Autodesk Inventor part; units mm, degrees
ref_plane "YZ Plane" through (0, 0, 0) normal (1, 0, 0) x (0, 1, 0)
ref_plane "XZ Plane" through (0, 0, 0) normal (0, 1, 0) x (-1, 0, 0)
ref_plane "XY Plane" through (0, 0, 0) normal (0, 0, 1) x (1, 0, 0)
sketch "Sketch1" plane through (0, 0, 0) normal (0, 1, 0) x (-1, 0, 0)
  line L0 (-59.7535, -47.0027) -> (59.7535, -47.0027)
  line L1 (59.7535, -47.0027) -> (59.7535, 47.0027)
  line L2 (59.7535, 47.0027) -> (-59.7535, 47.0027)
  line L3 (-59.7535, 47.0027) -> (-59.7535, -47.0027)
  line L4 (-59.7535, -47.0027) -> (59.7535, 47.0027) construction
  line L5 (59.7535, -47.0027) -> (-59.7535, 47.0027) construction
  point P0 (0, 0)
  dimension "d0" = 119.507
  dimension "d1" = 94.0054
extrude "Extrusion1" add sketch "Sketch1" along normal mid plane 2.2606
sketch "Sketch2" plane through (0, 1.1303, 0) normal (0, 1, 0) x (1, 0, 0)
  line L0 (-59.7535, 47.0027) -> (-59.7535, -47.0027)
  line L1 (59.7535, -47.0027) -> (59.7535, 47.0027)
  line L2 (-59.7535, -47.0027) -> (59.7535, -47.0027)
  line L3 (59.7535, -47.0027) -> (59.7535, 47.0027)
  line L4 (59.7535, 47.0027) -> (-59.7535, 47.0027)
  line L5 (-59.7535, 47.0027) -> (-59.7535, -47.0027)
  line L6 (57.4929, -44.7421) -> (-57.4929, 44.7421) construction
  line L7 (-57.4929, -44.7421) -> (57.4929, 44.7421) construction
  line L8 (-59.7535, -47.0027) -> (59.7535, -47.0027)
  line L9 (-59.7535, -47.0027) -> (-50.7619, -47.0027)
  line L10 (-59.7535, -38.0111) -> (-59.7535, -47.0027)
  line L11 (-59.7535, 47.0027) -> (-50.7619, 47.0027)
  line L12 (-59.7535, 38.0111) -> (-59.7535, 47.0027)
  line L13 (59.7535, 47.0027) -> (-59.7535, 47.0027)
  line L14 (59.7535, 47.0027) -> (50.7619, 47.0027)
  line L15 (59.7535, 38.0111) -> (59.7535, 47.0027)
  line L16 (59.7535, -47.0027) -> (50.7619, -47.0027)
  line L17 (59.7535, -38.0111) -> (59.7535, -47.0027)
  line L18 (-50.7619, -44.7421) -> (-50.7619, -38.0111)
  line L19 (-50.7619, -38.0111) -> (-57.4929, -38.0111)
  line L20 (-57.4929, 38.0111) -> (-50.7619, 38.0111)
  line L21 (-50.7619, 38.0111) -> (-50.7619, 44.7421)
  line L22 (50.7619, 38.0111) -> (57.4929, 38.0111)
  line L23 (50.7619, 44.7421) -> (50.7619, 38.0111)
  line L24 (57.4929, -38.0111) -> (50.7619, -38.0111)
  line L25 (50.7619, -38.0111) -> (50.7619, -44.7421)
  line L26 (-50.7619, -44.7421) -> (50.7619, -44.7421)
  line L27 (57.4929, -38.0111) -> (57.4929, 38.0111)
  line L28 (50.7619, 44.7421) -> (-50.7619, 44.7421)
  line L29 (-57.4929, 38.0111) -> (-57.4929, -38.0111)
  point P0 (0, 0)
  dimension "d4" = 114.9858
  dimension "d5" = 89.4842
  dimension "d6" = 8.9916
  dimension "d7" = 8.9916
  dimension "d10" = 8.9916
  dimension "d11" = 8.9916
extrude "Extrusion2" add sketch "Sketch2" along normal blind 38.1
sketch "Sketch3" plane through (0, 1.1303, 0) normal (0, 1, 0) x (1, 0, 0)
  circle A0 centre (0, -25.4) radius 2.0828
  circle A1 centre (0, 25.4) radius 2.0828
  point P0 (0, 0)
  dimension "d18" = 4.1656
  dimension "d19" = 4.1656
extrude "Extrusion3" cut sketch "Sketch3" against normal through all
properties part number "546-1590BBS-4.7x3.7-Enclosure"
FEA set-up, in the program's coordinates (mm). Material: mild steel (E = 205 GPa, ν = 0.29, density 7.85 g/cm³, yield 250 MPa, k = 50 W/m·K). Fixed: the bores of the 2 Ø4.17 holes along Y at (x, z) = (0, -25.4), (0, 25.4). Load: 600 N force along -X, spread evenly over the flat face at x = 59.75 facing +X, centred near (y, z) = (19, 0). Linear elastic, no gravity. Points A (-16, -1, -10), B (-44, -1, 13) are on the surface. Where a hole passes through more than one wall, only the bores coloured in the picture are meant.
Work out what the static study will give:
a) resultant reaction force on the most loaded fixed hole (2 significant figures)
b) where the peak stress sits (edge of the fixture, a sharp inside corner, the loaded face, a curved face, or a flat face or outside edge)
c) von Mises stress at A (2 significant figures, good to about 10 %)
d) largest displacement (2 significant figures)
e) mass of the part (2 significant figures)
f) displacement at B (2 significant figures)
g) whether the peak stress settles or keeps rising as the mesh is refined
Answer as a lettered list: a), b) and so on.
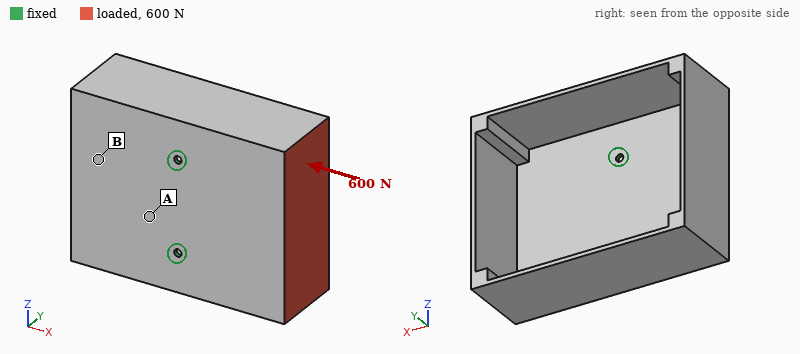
a) 300 N
b) edge of the fixture
c) 31 MPa
d) 0.42 mm
e) 540 g
f) 0.21 mm
g) keeps rising
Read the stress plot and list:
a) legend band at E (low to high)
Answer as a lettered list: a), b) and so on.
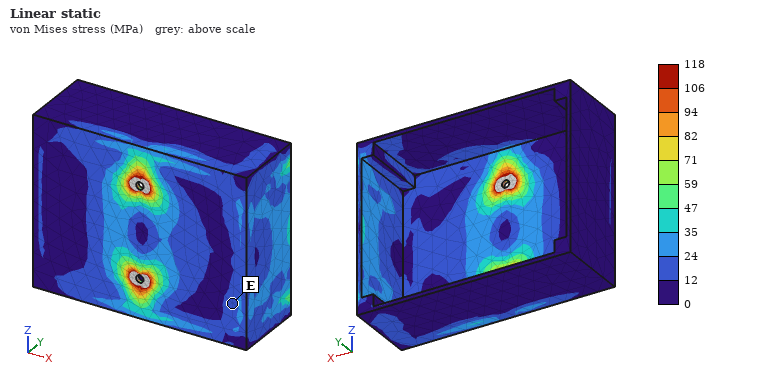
a) 12 to 24 MPa
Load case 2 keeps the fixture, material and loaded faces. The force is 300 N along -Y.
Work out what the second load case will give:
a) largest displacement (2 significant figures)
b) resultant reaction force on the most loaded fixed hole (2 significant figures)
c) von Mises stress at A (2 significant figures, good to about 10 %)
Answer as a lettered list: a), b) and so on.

a) 0.59 mm
b) 150 N
c) 41 MPa
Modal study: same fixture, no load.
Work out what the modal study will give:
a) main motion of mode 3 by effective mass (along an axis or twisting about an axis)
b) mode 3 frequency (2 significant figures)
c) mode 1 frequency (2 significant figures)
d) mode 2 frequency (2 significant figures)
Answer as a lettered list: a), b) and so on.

a) along Z
b) 670 Hz
c) 220 Hz
d) 450 Hz
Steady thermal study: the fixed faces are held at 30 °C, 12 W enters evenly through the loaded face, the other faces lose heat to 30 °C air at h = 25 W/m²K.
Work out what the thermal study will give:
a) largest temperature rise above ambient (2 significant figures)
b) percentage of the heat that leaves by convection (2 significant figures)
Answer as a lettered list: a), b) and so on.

a) 31 K
b) 78 %
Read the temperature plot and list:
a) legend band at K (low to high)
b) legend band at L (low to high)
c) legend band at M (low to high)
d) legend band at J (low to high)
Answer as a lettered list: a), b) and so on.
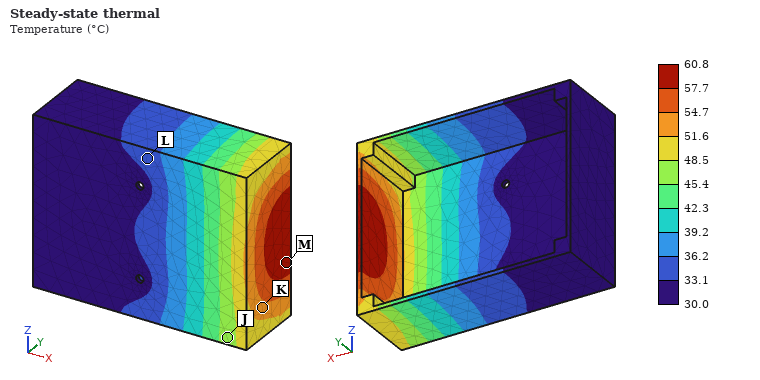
a) 51.6 to 54.7 °C
b) 33.1 to 36.2 °C
c) 57.7 to 60.8 °C
d) 45.4 to 48.5 °C
